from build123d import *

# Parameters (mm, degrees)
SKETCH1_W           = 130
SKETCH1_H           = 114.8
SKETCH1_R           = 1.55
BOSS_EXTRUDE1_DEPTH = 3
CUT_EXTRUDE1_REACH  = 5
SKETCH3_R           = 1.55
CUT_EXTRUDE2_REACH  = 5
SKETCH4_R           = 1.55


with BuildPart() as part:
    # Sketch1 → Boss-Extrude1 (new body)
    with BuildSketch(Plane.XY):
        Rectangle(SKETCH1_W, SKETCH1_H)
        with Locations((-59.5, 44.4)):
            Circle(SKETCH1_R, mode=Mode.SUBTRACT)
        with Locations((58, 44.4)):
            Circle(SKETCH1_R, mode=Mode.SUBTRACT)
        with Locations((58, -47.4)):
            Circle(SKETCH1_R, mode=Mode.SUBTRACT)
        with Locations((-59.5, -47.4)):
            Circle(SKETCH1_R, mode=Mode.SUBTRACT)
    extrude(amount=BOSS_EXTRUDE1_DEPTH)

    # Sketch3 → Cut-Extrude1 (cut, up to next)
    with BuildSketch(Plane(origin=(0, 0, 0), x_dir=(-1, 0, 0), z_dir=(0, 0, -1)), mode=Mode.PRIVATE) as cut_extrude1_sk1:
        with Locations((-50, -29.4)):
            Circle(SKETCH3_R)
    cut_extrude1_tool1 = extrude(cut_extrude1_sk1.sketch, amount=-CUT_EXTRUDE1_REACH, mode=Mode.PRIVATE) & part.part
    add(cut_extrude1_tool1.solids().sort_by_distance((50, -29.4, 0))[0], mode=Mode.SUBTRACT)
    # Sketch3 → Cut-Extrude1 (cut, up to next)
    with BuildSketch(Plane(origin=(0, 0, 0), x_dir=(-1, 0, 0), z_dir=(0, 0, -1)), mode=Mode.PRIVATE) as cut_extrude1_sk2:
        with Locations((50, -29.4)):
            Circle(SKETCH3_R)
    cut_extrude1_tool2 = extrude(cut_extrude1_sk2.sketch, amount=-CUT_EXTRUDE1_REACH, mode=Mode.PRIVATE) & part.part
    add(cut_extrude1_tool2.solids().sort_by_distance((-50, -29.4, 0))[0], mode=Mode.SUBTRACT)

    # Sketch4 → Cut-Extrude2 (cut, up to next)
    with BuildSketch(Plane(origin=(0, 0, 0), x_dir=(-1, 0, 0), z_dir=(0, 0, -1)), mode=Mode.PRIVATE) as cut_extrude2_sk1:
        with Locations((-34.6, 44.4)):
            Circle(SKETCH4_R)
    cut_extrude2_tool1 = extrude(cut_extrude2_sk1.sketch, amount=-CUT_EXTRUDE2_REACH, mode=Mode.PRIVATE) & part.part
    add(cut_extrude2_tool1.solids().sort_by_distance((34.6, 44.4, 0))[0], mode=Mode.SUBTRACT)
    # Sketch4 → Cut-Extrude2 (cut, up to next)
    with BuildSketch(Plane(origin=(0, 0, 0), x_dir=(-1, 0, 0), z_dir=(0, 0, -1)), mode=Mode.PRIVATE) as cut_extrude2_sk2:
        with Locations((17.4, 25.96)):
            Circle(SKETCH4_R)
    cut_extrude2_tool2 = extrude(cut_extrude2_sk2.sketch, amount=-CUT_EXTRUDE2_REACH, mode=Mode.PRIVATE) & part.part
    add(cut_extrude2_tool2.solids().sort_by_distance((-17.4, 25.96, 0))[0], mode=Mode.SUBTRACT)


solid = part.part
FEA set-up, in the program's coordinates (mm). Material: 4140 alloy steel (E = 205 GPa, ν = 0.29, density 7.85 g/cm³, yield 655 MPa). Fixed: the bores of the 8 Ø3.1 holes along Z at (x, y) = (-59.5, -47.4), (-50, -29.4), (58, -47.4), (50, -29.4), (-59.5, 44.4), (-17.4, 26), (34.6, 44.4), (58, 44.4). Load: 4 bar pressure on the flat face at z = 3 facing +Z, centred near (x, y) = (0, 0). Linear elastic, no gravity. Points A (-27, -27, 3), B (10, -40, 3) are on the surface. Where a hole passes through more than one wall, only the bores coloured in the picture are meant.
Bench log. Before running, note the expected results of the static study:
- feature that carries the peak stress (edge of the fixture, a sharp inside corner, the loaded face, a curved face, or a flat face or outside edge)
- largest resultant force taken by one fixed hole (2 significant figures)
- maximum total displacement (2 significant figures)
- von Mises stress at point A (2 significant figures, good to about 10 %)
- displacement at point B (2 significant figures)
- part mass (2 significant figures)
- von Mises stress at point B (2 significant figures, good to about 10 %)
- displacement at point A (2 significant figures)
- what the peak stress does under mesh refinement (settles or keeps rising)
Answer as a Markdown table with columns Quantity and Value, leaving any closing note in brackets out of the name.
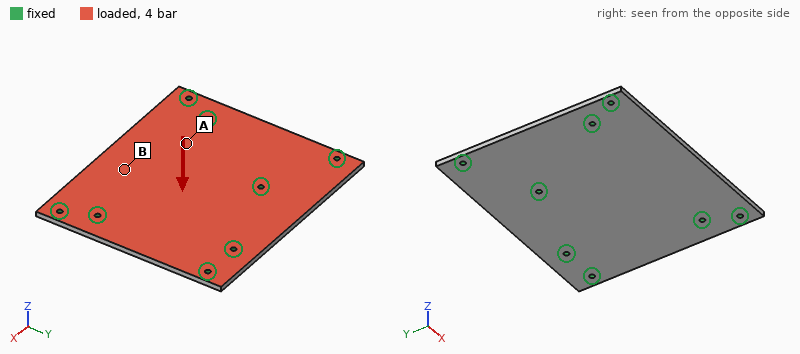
| Quantity | Value |
|---|---|
| feature that carries the peak stress | edge of the fixture |
| largest resultant force taken by one fixed hole | 1.5 kN |
| maximum total displacement | 0.33 mm |
| von Mises stress at point A | 58 MPa |
| displacement at point B | 0.25 mm |
| part mass | 350 g |
| von Mises stress at point B | 100 MPa |
| displacement at point A | 0.13 mm |
| what the peak stress does under mesh refinement | keeps rising |
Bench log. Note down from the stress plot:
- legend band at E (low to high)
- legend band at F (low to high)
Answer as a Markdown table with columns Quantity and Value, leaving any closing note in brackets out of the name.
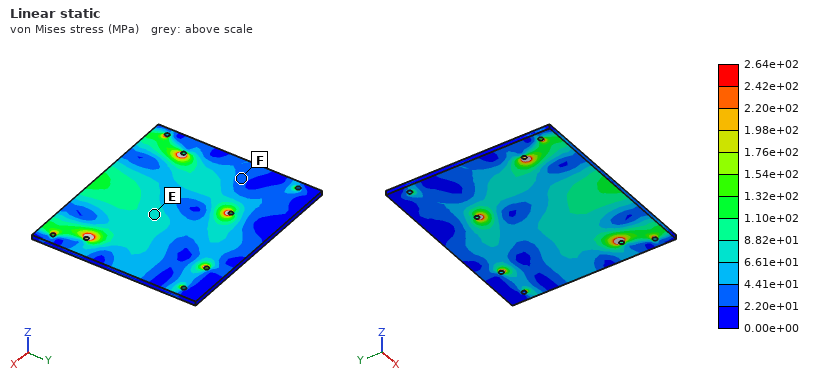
| Quantity | Value |
|---|---|
| legend band at E | 6.61e+01 to 8.82e+01 MPa |
| legend band at F | 2.20e+01 to 4.41e+01 MPa |
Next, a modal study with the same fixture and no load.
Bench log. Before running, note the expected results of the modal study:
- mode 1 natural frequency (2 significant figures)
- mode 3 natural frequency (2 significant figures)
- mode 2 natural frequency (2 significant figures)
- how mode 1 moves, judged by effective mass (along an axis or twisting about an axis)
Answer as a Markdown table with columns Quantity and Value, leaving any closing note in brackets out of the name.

| Quantity | Value |
|---|---|
| mode 1 natural frequency | 1500 Hz |
| mode 3 natural frequency | 2900 Hz |
| mode 2 natural frequency | 2400 Hz |
| how mode 1 moves, judged by effective mass | along Z |
